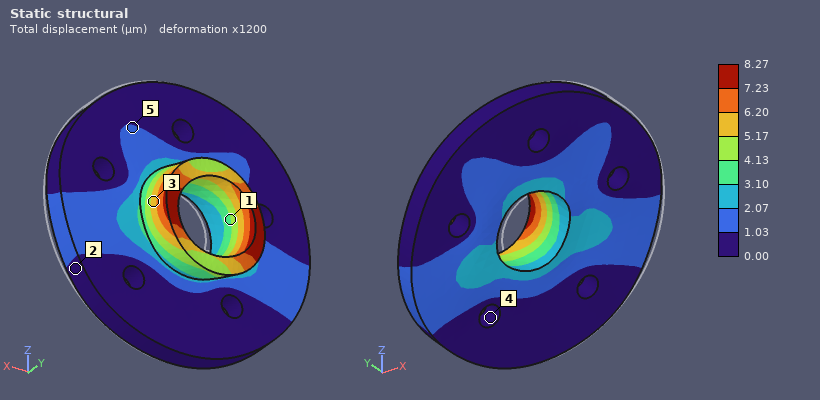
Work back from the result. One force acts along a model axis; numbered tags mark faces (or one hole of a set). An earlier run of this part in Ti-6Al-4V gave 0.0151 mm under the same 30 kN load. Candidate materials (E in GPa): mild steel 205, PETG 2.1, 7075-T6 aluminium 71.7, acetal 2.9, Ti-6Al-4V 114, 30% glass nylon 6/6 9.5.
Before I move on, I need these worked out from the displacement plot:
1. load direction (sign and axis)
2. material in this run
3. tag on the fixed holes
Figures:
-X
mild steel
4
